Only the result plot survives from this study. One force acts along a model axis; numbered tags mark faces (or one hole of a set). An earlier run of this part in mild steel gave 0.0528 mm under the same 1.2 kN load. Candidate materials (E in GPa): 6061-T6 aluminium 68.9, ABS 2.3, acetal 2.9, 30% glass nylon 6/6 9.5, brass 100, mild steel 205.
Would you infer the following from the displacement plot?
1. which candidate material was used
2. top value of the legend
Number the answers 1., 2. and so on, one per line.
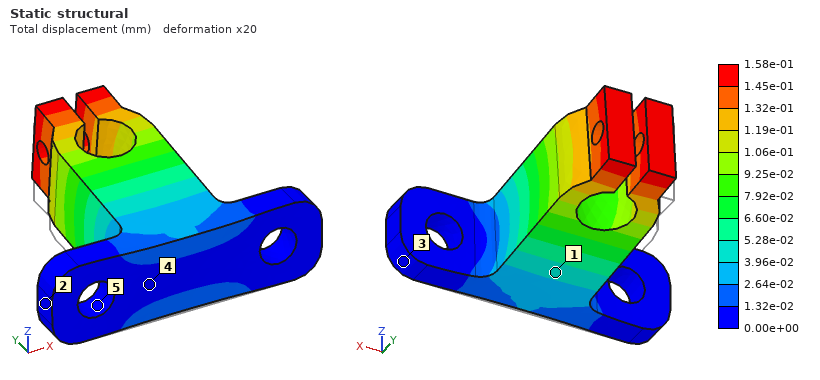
1. 6061-T6 aluminium
2. 1.58e-01 mm
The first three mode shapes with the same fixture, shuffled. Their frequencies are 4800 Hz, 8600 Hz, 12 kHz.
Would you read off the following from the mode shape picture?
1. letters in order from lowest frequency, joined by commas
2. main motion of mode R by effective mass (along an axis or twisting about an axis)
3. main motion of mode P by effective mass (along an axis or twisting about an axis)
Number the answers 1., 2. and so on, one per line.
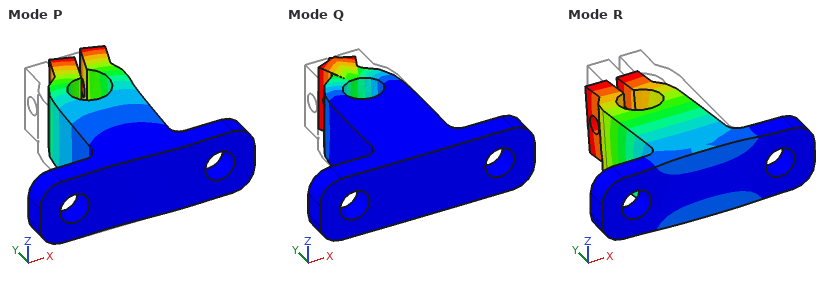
1. R, P, Q
2. along Z
3. along X
